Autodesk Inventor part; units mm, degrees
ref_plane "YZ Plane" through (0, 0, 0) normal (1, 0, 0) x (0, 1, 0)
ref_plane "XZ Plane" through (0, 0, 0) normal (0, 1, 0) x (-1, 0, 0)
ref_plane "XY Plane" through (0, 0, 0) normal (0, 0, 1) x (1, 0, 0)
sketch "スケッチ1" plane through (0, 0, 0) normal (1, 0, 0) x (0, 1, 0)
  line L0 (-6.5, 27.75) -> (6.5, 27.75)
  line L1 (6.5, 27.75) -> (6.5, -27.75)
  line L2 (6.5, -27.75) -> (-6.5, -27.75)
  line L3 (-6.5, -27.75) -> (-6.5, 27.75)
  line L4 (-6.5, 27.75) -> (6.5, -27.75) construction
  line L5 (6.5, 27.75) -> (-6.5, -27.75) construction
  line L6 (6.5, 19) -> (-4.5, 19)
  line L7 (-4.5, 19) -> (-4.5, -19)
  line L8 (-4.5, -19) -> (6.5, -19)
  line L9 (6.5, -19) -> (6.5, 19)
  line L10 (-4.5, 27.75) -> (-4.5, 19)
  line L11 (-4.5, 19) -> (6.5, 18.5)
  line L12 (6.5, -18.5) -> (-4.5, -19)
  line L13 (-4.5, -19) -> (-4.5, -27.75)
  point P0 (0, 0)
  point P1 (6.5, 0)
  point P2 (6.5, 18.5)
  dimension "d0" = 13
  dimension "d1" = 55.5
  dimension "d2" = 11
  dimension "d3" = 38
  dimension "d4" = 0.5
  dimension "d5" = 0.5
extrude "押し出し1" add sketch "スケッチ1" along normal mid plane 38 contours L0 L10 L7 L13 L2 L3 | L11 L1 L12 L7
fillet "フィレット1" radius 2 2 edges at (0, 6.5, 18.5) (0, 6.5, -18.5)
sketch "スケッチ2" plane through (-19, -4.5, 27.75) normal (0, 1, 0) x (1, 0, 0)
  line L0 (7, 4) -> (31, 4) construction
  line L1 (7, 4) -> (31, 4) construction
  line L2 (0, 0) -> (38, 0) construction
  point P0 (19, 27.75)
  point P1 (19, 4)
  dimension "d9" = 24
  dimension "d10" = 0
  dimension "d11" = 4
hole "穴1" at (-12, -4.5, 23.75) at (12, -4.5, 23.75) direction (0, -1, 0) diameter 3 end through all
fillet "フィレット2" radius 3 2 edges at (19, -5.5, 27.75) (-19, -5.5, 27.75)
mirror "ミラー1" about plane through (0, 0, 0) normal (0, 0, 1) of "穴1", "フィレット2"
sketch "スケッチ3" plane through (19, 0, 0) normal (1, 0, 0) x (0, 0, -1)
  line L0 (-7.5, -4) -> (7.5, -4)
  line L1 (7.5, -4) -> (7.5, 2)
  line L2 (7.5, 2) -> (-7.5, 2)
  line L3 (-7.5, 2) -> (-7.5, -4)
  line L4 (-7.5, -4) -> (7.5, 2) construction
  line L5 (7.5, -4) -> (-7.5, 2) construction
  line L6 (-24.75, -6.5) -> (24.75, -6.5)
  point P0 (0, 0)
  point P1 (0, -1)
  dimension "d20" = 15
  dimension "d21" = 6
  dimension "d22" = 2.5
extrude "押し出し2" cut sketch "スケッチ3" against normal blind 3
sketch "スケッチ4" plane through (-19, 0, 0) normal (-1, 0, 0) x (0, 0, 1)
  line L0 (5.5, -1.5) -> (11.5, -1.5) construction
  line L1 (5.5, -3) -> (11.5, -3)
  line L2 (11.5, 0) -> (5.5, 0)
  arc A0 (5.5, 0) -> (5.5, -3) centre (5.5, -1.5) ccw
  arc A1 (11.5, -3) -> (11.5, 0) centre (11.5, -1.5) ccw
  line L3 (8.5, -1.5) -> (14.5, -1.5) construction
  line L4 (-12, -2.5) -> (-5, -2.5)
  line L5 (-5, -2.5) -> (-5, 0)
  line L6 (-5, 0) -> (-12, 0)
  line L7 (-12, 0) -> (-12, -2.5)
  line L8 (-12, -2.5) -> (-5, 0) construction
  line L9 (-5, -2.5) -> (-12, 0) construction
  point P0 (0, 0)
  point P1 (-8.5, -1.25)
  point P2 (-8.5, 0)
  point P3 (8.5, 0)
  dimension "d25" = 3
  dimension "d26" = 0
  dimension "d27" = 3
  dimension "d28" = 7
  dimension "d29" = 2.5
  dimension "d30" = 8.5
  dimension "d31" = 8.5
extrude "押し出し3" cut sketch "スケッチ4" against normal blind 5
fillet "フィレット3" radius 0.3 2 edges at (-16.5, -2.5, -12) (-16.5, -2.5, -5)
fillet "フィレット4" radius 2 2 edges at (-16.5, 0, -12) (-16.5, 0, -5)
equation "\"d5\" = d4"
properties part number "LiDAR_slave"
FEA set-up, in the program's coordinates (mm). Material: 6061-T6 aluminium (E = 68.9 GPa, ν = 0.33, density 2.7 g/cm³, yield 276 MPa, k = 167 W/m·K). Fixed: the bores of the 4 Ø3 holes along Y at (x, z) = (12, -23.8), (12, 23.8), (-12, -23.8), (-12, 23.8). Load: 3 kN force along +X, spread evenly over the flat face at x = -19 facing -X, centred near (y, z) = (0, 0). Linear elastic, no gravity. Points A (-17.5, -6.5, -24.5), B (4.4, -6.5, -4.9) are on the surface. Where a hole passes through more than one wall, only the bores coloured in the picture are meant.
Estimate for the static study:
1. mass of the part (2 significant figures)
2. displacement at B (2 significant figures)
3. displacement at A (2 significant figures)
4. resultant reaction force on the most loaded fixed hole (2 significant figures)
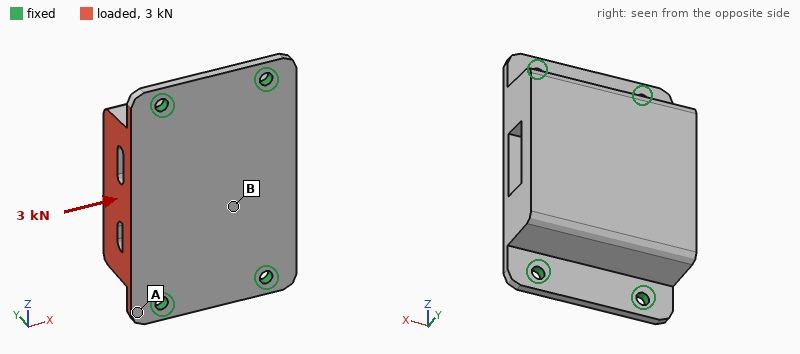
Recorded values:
52 g
8.0 µm
5.5 µm
920 N
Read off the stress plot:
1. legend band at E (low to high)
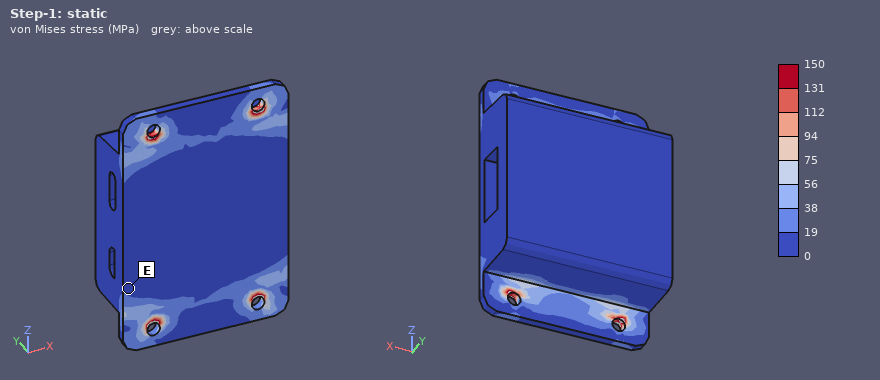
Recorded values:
0 to 19 MPa
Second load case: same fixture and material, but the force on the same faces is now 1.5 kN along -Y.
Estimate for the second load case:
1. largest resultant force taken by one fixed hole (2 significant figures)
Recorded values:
1.1 kN
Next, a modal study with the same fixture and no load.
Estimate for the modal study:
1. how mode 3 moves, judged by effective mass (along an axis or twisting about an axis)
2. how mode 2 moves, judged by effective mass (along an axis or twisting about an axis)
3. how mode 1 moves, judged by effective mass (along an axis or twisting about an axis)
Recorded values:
along Z
along Y
along X
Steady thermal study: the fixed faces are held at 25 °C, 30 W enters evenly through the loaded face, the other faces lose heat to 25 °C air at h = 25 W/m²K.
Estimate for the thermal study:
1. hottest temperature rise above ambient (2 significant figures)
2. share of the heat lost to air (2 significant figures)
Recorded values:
16 K
4.5 %
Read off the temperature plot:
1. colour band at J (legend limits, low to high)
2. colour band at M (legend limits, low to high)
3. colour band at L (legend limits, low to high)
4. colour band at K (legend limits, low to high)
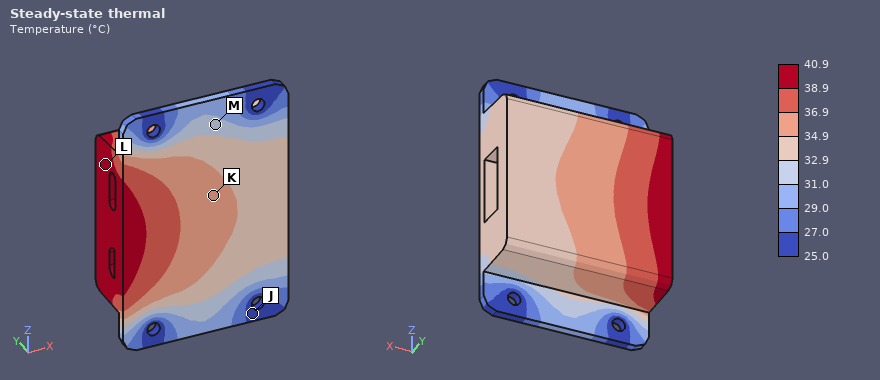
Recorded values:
25.0 to 27.0 °C
31.0 to 32.9 °C
38.9 to 40.9 °C
34.9 to 36.9 °C
